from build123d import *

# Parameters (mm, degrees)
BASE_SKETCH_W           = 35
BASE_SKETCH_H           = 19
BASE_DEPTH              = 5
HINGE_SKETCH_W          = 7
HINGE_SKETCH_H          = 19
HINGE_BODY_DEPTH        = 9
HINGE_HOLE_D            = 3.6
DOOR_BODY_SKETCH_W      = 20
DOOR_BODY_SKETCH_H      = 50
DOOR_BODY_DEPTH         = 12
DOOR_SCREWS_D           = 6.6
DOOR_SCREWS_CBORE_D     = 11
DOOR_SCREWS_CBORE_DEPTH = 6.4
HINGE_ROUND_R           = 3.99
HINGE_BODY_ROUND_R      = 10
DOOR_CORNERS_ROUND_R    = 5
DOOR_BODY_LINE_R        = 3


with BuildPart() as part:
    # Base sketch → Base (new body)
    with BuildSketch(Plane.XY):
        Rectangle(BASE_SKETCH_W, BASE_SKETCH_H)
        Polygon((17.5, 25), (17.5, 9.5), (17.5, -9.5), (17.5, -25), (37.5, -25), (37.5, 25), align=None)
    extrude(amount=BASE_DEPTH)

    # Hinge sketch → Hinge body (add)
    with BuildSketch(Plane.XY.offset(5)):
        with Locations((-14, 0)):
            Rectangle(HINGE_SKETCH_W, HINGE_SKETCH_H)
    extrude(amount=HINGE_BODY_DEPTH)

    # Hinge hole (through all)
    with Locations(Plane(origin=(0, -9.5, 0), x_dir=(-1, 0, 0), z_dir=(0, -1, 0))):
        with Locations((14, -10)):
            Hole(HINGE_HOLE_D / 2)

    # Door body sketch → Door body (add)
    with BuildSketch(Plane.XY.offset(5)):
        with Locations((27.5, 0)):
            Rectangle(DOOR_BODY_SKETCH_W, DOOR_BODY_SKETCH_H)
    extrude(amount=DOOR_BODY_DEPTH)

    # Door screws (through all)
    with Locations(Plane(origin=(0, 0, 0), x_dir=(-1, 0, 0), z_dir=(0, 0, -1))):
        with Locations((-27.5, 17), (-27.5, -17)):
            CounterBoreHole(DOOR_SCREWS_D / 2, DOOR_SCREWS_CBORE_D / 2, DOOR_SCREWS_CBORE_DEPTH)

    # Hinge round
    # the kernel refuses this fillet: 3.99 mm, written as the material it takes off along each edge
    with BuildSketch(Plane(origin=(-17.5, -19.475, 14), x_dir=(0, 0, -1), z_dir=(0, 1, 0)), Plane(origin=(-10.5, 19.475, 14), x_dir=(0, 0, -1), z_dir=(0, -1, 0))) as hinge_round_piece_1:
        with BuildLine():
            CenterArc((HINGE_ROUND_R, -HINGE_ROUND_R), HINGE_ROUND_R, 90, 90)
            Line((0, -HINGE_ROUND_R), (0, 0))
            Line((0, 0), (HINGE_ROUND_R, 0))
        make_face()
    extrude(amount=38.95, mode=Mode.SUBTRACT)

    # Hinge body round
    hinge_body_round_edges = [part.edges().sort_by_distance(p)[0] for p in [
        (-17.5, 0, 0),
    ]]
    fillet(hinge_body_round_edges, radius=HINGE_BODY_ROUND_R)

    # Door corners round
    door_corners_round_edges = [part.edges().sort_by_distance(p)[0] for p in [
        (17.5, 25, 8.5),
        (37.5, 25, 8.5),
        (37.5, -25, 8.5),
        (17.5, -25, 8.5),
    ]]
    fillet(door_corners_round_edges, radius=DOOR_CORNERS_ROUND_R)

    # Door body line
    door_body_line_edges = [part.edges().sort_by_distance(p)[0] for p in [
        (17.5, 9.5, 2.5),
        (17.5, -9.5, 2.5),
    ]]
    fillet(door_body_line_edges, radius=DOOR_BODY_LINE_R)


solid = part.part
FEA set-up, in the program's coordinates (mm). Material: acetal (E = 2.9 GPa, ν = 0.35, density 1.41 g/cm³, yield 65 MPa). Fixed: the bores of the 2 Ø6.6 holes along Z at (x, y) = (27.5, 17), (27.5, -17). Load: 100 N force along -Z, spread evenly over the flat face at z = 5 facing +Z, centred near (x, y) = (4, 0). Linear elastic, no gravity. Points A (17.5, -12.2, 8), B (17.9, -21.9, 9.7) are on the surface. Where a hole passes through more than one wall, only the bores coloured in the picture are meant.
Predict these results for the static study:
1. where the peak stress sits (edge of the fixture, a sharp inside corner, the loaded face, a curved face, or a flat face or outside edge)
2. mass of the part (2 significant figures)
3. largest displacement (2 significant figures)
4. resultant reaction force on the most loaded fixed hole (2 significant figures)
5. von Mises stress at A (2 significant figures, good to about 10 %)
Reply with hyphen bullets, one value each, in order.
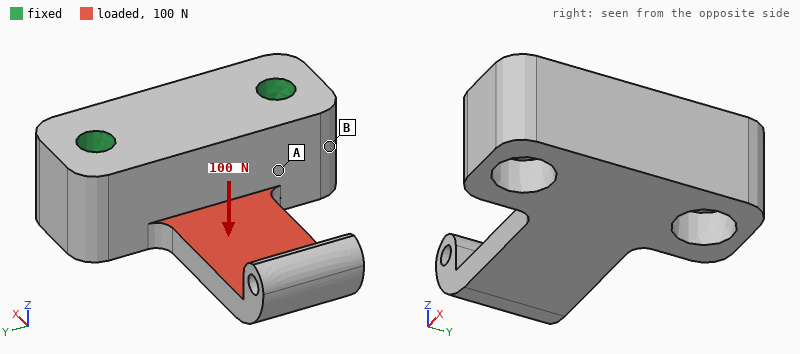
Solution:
- a curved face
- 26 g
- 0.91 mm
- 60 N
- 2.6 MPa
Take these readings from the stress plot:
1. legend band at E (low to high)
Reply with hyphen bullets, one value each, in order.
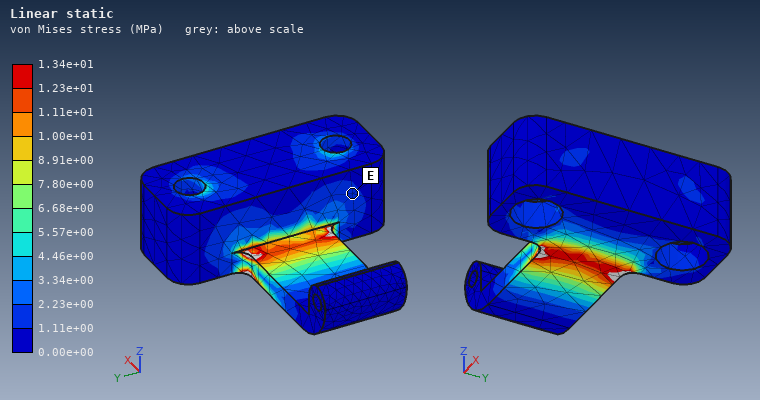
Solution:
- 1.11e+00 to 2.23e+00 MPa
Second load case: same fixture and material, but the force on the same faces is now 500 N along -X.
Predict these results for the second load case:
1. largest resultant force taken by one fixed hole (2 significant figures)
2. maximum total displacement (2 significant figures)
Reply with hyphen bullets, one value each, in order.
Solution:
- 250 N
- 0.83 mm
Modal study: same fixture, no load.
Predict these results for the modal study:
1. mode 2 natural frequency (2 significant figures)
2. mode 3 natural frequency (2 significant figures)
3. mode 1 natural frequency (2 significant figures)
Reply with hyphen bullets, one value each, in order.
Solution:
- 1800 Hz
- 2900 Hz
- 690 Hz
